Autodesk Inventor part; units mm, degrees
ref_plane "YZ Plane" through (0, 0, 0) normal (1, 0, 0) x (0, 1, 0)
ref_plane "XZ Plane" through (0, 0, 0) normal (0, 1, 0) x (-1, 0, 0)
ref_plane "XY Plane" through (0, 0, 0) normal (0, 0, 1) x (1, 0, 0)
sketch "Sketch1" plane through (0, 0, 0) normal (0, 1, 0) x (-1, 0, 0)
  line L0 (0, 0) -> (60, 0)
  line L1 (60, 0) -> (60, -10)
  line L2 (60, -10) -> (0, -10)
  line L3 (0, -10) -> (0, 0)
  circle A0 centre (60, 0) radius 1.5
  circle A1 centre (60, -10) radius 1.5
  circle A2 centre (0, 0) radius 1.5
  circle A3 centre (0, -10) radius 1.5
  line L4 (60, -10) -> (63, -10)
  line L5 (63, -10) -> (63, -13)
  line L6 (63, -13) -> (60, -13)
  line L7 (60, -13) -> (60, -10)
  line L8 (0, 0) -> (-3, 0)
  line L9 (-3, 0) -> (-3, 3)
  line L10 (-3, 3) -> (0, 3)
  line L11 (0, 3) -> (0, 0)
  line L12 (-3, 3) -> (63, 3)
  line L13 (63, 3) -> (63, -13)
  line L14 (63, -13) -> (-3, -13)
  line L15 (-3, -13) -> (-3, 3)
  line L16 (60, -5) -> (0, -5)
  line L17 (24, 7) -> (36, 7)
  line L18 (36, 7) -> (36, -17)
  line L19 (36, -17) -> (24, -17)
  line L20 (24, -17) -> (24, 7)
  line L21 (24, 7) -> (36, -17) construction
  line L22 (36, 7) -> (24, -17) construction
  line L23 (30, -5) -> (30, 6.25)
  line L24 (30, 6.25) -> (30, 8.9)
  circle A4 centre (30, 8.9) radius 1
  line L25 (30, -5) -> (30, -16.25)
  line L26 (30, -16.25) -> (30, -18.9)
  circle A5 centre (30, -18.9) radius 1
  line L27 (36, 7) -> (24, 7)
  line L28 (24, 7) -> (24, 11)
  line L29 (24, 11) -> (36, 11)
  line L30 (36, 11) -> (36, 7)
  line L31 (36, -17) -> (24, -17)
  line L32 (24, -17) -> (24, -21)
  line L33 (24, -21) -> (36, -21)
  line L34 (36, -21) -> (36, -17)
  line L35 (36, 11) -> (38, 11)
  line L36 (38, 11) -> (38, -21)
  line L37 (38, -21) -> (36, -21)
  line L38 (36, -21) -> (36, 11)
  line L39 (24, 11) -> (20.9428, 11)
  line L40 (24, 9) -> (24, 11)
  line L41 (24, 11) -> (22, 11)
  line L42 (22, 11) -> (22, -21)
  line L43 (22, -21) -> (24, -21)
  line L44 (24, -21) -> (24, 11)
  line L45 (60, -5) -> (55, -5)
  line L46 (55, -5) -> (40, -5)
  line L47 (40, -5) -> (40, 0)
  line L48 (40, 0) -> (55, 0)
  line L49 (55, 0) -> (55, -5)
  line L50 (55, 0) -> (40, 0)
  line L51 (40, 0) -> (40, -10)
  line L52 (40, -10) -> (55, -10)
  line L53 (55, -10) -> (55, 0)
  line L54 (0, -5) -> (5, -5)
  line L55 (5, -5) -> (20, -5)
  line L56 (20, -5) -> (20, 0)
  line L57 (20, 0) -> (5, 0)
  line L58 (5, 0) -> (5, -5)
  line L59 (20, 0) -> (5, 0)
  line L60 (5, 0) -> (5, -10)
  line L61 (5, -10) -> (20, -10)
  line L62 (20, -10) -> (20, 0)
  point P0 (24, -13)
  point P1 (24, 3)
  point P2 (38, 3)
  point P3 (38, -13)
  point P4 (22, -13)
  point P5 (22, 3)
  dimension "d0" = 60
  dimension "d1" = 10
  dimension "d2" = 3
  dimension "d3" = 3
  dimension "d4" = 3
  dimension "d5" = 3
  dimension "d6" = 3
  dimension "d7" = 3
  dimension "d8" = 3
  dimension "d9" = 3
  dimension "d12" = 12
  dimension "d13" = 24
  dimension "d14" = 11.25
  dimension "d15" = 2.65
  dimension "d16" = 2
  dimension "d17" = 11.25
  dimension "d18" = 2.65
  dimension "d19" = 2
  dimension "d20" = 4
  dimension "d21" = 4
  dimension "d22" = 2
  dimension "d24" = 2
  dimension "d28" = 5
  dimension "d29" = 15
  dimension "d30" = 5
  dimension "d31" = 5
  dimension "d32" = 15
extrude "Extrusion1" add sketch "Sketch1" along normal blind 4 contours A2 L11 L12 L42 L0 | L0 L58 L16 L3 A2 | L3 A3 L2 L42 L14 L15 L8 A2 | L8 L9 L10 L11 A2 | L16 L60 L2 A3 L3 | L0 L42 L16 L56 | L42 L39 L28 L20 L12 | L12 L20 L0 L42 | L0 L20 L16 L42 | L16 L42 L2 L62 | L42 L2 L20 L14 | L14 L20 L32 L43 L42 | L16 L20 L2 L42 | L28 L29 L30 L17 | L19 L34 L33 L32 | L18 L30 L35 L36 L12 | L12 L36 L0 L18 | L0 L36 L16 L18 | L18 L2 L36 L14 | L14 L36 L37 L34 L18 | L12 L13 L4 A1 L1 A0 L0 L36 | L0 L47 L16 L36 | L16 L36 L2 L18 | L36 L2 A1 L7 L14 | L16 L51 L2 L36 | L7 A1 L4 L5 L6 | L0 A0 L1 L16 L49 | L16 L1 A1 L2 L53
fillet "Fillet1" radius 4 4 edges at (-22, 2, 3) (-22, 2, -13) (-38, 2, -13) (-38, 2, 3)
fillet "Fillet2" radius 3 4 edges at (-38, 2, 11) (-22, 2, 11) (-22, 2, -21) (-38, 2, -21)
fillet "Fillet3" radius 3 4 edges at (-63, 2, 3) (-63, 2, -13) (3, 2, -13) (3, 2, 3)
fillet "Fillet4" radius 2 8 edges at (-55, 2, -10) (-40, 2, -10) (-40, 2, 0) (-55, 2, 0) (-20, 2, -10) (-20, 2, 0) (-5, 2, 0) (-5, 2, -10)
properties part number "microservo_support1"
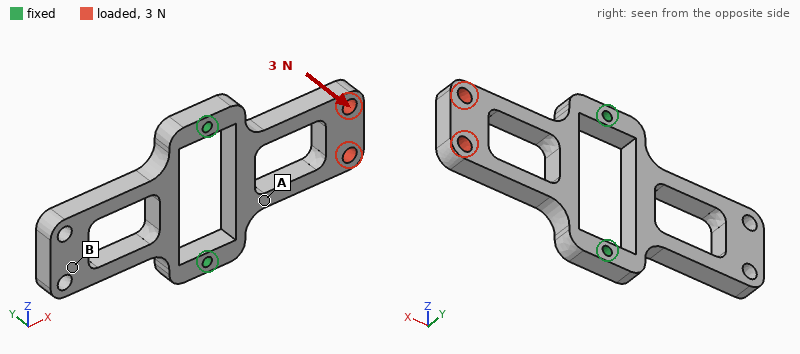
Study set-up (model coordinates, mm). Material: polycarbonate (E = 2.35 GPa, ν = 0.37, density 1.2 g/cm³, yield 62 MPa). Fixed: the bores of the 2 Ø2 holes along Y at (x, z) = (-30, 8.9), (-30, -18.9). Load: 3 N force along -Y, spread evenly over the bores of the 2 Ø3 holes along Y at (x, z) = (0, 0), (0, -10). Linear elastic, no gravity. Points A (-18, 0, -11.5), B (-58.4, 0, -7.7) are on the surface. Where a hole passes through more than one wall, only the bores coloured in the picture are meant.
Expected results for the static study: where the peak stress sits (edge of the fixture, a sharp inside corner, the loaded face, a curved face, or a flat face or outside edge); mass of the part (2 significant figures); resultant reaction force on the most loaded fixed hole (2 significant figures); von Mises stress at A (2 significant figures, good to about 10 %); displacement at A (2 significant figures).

a flat face or outside edge
3.3 g
1.5 N
3.2 MPa
0.13 mm
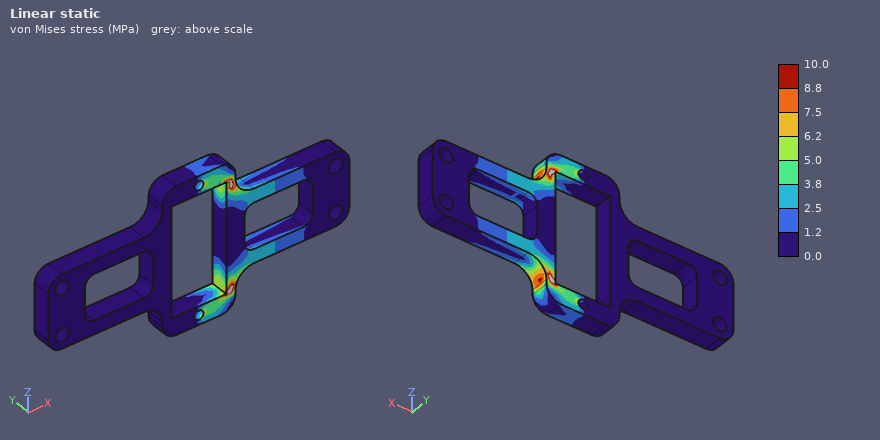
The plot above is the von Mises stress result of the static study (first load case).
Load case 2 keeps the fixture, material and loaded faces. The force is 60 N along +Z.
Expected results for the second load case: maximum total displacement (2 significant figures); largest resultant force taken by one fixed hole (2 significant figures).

0.79 mm
68 N
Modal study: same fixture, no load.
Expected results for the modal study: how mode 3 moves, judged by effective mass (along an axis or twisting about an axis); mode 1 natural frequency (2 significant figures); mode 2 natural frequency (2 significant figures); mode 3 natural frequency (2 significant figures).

twisting about Y
470 Hz
470 Hz
1800 Hz
